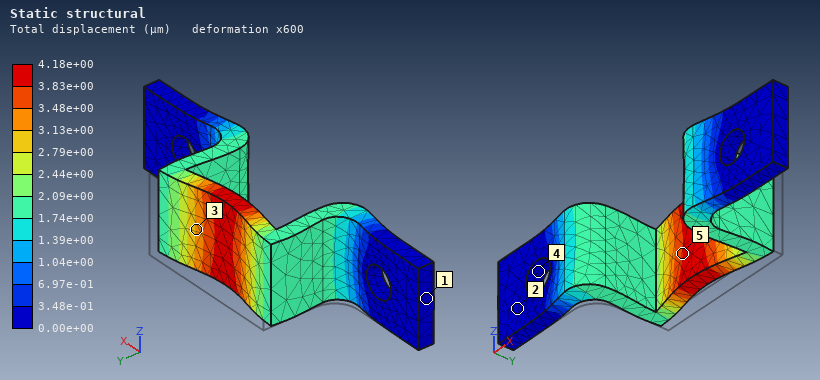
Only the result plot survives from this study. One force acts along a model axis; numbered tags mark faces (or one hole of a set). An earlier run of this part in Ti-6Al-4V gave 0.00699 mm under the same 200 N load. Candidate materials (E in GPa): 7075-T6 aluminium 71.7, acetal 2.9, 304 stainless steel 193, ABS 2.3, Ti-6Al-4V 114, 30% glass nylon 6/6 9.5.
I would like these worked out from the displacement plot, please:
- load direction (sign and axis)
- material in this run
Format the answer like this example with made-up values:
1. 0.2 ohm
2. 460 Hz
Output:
1. -Y
2. 304 stainless steel
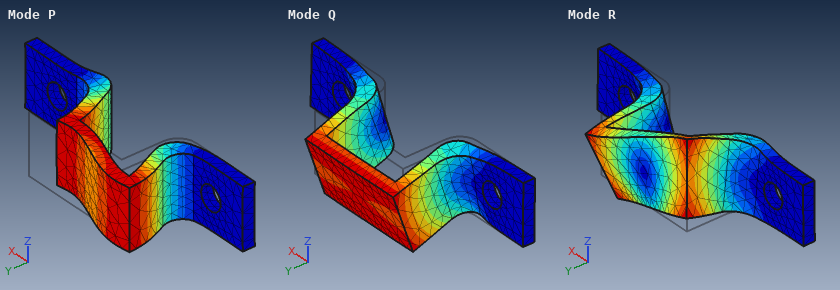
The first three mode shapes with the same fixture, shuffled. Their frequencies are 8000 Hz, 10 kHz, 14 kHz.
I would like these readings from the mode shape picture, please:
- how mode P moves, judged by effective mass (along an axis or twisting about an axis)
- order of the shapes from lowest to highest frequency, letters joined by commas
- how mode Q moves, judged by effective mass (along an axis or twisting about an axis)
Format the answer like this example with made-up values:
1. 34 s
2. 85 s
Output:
1. along X
2. Q, P, R
3. along Z
